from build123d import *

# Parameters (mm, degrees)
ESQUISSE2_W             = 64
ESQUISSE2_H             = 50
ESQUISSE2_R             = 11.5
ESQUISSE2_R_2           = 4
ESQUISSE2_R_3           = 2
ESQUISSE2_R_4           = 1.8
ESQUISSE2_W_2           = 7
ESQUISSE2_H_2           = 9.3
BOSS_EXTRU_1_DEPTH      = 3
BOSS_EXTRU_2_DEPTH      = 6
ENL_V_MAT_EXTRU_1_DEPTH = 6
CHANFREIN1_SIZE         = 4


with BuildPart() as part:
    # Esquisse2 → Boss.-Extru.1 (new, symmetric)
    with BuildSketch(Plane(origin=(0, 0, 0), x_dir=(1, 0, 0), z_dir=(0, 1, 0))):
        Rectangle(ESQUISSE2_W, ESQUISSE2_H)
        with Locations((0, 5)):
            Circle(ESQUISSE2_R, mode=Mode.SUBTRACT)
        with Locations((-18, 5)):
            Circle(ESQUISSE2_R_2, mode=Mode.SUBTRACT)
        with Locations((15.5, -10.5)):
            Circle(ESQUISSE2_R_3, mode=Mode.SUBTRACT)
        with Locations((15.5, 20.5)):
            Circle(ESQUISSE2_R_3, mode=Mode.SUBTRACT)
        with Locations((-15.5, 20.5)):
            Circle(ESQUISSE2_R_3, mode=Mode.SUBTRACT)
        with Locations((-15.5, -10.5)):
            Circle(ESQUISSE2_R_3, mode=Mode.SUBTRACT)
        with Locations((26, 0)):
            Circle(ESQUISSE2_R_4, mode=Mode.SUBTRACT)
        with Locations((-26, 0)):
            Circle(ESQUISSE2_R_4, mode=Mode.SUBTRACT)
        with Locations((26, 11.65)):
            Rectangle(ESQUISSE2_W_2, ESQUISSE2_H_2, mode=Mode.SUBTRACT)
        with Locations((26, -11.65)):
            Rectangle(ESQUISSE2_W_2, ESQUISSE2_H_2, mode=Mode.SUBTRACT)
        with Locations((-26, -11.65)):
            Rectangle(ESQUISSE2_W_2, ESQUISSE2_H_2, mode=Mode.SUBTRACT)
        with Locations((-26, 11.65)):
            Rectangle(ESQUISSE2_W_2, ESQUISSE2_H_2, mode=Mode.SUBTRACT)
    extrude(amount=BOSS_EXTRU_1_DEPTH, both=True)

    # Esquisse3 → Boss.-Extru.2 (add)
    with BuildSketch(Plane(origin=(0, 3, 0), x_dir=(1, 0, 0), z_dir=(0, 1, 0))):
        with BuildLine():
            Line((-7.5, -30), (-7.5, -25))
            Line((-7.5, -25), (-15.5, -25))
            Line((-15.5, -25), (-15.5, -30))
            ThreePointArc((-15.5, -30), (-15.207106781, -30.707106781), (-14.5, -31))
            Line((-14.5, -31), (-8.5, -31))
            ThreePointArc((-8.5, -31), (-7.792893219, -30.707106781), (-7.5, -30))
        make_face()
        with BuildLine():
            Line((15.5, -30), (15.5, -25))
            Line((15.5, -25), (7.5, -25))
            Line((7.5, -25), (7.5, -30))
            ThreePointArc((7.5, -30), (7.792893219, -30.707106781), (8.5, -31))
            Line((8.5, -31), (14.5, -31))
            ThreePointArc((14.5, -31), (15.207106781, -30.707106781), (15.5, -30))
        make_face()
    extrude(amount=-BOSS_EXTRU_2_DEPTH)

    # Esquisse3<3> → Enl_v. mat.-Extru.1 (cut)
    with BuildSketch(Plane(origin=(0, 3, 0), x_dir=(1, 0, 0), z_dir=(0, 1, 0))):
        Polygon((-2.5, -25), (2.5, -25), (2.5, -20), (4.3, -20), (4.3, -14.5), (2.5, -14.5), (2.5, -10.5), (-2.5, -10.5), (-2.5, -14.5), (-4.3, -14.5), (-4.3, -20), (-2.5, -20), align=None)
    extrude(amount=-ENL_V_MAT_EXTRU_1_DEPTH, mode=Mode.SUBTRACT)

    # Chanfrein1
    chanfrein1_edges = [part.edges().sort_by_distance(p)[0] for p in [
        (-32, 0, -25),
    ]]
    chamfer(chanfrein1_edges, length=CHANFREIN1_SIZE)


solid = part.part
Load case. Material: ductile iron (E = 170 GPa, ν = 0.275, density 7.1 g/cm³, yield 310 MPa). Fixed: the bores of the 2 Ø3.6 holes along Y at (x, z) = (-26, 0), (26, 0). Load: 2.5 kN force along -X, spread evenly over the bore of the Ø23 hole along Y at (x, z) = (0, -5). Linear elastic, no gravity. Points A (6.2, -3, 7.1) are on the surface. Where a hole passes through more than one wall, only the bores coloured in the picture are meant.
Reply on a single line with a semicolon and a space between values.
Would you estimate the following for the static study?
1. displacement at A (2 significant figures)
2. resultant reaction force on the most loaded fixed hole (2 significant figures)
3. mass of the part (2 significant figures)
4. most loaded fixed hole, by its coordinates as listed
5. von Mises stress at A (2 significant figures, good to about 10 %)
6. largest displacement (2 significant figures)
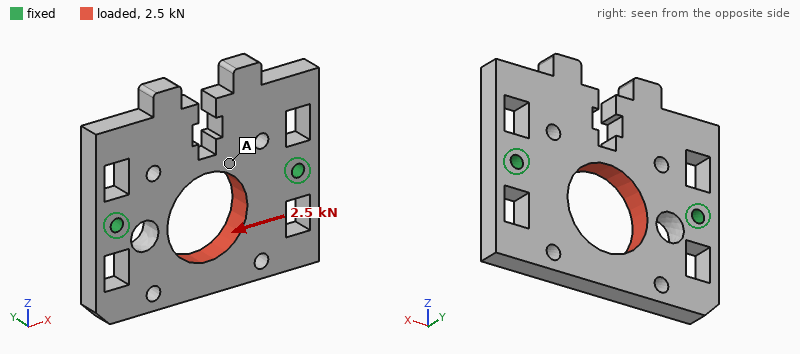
1.3 µm; 1.4 kN; 100 g; (26, 0); 7.2 MPa; 5.7 µm
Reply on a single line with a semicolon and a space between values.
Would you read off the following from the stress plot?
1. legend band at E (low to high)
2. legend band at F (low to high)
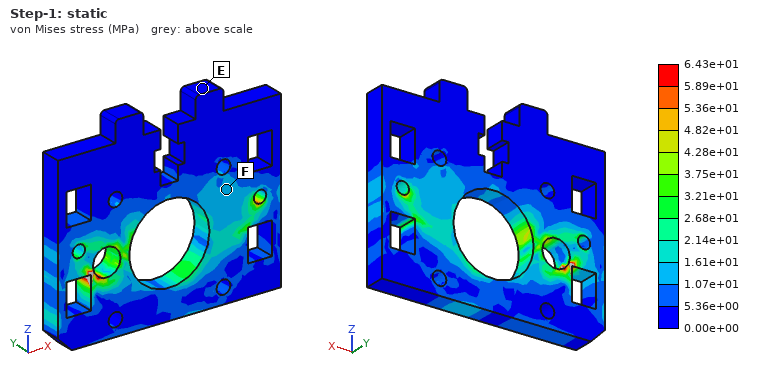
0.00e+00 to 5.36e+00 MPa; 1.07e+01 to 1.61e+01 MPa
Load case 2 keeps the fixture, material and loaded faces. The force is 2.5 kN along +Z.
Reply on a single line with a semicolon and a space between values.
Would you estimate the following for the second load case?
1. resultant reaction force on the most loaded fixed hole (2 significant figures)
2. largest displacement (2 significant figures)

1.3 kN; 9.6 µm
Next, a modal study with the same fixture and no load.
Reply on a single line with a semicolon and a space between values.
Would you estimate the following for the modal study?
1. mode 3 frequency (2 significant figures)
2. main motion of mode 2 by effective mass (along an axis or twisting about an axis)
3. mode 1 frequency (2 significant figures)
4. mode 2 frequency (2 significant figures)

5300 Hz; along Y; 3500 Hz; 4500 Hz
